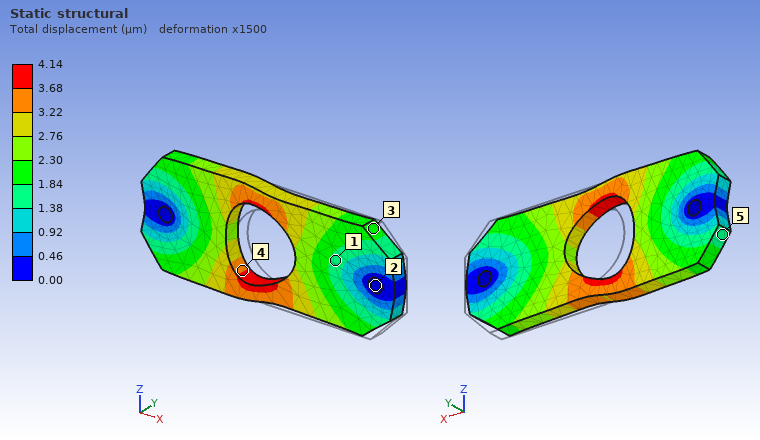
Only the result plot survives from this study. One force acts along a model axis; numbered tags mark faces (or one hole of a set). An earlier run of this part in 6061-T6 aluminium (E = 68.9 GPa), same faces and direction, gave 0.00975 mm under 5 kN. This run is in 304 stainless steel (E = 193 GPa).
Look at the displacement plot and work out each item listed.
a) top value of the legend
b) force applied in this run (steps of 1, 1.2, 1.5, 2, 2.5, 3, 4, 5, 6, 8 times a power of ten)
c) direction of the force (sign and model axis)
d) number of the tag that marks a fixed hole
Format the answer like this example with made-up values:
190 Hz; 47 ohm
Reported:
4.14 µm; 6 kN; -X; 2
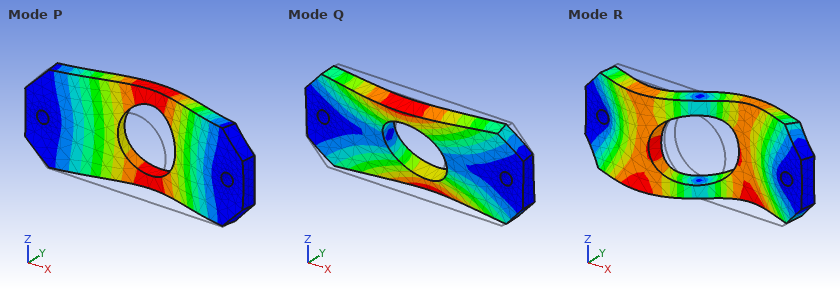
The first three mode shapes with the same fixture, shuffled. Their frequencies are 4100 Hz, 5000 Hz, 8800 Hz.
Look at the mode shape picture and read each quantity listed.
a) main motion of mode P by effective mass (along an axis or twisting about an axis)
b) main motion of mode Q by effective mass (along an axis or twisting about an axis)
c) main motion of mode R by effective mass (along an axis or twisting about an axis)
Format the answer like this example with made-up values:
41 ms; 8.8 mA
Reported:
along Y; twisting about X; twisting about Z
